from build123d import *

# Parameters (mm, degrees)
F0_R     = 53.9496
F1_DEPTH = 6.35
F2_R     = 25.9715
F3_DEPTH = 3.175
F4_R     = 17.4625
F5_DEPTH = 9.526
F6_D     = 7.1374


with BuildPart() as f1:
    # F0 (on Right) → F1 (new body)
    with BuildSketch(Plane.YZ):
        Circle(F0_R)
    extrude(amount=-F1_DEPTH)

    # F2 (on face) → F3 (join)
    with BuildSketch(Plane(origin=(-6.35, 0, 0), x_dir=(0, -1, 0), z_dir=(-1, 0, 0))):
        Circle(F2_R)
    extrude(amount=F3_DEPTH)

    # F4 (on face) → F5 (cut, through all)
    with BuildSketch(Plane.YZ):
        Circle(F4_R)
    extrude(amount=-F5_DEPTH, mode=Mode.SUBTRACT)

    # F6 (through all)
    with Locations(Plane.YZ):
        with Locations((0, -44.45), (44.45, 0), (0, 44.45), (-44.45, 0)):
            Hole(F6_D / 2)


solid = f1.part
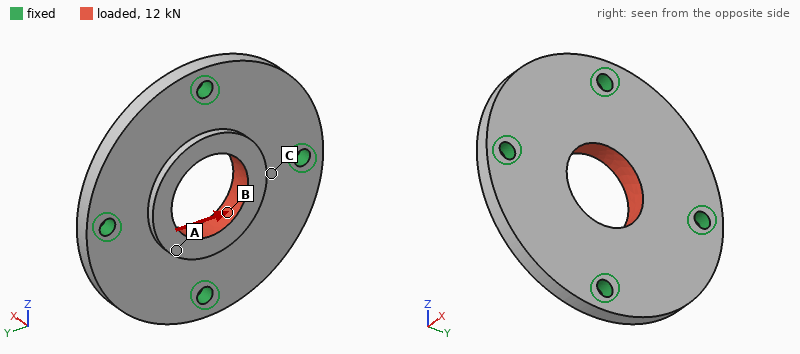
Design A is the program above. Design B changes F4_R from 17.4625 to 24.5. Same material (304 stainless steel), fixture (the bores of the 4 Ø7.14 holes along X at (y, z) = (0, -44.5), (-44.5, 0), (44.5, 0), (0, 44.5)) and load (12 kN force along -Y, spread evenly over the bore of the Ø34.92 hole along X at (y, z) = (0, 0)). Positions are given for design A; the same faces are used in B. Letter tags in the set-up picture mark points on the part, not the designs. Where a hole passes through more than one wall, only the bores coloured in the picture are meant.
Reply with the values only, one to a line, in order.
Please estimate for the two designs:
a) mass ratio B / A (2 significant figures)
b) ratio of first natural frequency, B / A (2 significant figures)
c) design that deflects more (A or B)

0.84
0.97
B
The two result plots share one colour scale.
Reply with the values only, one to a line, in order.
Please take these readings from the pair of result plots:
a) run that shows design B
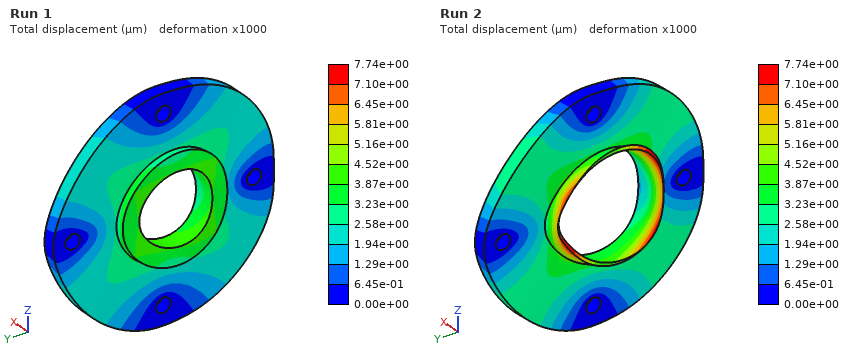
Run 2
